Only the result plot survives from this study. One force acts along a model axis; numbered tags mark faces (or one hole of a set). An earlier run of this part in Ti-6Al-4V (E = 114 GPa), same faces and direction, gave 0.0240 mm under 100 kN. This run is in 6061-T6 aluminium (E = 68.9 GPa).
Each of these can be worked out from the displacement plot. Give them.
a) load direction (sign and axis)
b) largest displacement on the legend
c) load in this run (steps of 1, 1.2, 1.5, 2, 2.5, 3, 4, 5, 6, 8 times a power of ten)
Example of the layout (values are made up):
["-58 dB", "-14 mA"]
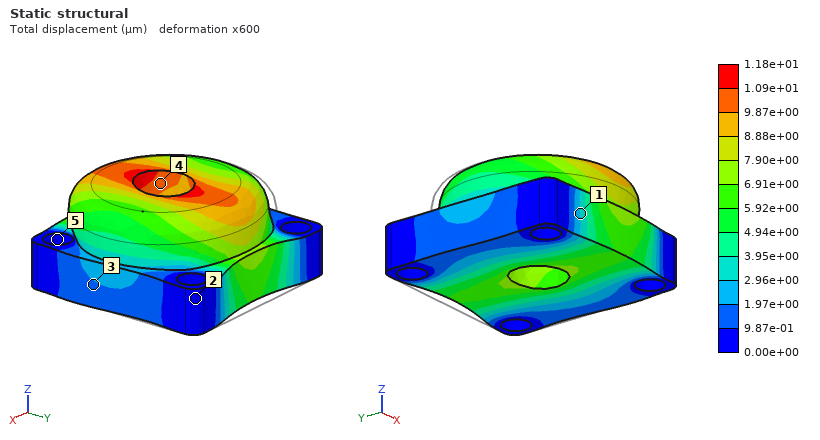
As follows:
["-Y", "1.18e+01 µm", "30 kN"]
